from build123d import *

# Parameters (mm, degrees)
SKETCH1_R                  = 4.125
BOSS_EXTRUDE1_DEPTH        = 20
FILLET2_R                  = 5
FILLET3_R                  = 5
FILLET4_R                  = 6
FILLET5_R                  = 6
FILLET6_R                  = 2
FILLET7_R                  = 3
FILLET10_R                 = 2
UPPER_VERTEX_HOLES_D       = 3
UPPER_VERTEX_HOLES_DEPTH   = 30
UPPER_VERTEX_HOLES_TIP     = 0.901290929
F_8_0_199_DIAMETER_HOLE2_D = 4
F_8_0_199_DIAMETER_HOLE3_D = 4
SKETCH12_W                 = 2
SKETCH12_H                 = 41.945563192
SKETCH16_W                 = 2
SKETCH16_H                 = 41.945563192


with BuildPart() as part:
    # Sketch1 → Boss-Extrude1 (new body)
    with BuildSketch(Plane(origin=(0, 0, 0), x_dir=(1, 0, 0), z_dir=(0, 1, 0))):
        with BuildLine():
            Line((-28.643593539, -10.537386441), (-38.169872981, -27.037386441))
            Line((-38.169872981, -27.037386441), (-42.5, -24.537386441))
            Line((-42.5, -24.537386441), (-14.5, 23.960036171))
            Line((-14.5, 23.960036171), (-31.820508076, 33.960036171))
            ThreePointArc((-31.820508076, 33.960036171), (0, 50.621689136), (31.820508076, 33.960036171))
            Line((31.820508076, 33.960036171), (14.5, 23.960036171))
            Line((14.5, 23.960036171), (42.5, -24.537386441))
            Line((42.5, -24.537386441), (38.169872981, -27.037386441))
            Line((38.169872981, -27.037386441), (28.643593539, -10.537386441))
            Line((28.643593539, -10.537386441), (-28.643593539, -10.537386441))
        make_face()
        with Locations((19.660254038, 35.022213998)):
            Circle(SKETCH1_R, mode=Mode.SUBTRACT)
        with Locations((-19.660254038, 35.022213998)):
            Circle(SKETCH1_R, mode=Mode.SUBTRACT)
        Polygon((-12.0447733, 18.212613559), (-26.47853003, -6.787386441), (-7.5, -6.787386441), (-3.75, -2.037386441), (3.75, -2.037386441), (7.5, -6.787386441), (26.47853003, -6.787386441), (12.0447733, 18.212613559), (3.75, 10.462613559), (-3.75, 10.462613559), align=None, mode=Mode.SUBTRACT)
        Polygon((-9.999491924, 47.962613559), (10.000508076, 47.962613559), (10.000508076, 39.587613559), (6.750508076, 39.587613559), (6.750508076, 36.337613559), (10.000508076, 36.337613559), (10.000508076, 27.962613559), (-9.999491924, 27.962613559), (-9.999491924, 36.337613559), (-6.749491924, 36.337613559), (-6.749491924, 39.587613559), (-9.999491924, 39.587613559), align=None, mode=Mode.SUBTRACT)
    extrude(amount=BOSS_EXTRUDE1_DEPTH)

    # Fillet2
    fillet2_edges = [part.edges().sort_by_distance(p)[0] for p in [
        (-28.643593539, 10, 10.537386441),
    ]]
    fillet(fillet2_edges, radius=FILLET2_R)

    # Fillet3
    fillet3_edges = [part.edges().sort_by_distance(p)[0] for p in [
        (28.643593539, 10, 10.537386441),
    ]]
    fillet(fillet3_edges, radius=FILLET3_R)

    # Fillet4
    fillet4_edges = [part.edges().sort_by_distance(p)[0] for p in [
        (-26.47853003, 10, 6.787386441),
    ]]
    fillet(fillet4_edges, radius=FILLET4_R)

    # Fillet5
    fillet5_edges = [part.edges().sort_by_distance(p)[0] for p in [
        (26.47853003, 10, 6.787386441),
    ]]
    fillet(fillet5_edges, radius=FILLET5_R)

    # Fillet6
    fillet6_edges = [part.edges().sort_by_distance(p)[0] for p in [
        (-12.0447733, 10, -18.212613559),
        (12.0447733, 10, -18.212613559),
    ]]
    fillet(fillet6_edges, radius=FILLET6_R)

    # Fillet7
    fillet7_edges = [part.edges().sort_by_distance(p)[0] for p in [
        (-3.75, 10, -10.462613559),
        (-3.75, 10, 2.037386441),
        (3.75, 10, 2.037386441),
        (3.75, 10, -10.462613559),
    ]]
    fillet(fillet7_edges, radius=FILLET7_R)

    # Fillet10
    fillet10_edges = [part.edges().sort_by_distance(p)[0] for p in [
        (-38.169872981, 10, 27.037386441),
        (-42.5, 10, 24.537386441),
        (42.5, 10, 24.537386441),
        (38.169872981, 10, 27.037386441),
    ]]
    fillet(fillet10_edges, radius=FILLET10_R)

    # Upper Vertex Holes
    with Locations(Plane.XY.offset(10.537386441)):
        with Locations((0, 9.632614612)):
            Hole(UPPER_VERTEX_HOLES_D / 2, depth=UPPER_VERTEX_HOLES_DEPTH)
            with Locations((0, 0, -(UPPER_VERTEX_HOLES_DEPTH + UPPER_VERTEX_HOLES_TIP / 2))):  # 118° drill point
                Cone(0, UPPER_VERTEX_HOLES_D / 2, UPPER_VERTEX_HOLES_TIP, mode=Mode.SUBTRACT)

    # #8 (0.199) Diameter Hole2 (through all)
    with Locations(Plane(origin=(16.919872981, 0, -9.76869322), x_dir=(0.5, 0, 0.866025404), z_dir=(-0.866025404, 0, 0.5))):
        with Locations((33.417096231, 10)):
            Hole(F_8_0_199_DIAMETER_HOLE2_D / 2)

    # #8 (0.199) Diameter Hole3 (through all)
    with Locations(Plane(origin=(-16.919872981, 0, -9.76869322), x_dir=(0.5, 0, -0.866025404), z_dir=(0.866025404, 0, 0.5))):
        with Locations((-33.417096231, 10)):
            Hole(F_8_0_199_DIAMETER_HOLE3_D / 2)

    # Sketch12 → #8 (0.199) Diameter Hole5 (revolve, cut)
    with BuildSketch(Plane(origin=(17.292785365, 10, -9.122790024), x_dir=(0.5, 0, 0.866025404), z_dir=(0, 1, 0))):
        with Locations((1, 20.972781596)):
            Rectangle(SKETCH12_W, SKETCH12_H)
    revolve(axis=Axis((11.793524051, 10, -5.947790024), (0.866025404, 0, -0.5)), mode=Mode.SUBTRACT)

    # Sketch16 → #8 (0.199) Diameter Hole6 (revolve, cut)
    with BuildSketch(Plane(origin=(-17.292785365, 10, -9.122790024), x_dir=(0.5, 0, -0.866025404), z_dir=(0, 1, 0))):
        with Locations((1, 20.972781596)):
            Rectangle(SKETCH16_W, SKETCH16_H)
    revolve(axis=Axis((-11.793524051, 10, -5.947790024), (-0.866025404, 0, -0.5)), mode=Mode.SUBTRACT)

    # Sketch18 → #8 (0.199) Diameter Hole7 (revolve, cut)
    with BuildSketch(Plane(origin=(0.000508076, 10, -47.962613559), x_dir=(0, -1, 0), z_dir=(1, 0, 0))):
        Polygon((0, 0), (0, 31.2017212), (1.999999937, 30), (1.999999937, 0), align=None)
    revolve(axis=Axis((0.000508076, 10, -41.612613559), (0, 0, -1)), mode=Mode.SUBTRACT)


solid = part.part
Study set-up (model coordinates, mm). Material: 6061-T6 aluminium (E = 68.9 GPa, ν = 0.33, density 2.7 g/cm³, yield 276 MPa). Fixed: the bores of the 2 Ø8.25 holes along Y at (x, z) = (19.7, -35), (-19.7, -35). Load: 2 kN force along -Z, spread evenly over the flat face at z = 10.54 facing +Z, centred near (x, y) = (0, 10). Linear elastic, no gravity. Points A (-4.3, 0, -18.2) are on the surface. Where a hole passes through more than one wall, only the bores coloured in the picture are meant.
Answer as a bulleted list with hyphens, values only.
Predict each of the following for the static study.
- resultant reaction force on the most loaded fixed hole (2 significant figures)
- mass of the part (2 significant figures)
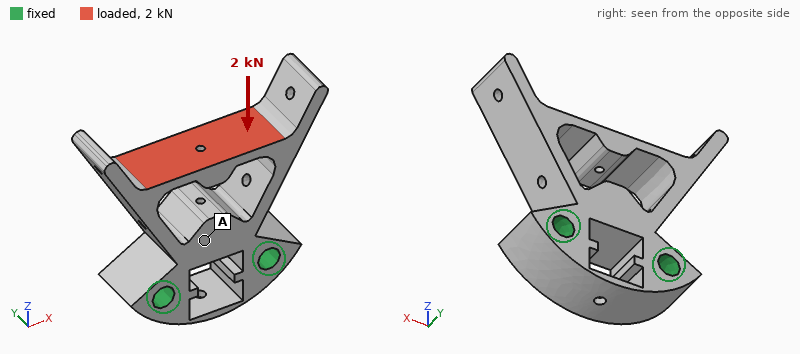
- 1.0 kN
- 99 g
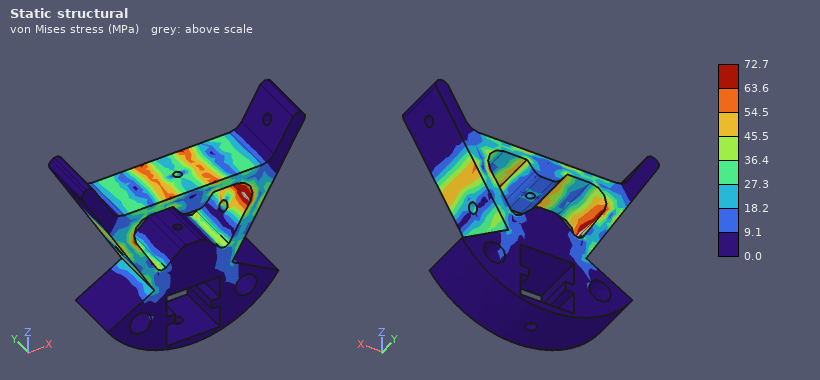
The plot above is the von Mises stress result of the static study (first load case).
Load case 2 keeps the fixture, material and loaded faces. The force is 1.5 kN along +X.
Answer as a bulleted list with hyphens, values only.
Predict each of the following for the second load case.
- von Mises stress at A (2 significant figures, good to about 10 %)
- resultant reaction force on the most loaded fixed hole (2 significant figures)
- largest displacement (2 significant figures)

- 16 MPa
- 2.1 kN
- 0.56 mm
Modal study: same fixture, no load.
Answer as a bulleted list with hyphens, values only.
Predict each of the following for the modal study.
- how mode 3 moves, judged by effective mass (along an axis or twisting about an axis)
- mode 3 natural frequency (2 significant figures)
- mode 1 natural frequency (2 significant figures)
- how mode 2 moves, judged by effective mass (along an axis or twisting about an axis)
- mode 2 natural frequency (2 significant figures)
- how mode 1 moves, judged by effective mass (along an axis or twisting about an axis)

- twisting about Z
- 3800 Hz
- 1700 Hz
- along Y
- 3000 Hz
- along X
